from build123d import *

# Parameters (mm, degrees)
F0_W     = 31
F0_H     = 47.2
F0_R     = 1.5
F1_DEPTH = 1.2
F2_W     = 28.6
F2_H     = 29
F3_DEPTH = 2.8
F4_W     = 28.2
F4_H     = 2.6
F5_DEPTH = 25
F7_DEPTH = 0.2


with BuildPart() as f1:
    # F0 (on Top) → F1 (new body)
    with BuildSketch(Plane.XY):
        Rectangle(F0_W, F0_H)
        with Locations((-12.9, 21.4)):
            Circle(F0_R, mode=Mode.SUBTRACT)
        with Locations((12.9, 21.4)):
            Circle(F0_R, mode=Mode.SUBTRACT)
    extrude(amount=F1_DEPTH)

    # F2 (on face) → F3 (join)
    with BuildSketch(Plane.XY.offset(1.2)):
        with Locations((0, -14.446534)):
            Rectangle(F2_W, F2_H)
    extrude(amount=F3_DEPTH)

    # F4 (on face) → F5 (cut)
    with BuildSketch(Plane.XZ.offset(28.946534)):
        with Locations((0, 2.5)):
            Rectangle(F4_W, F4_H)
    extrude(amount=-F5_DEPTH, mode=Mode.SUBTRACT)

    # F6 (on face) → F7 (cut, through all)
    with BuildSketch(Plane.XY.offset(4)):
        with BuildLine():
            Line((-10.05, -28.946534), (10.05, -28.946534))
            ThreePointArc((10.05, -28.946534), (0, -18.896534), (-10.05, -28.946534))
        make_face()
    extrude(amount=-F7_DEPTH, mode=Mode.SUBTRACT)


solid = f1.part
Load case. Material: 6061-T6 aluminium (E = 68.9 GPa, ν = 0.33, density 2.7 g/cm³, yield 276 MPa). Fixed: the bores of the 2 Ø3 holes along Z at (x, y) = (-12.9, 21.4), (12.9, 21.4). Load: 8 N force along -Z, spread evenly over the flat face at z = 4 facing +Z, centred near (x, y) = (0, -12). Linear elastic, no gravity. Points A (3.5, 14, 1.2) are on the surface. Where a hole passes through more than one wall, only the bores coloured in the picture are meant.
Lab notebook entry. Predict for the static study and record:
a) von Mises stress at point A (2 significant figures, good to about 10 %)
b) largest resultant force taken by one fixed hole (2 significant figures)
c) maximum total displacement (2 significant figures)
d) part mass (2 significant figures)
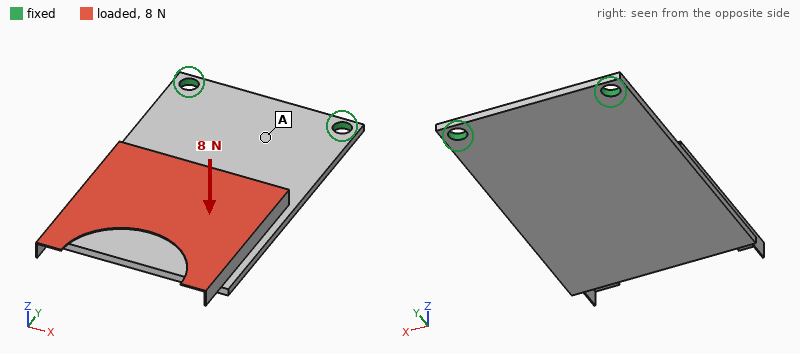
22 MPa
4.0 N
0.66 mm
5.9 g
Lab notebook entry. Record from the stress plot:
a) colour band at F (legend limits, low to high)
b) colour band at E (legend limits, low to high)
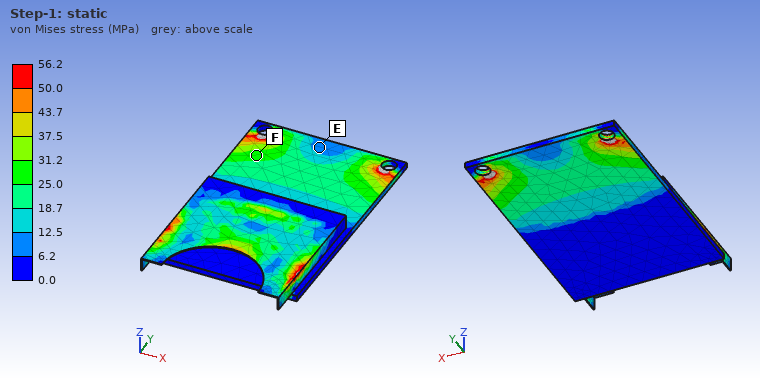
25.0 to 31.2 MPa
6.2 to 12.5 MPa
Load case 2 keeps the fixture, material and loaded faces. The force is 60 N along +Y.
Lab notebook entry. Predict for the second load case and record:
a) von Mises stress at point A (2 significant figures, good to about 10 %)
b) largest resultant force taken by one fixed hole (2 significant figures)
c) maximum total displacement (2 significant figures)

23 MPa
31 N
0.61 mm
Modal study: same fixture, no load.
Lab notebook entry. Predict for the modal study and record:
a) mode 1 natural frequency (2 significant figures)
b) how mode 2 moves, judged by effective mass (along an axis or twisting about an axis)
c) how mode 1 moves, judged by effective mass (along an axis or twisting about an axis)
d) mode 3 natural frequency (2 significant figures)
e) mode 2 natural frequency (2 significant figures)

420 Hz
twisting about Y
along Z
2200 Hz
1800 Hz
